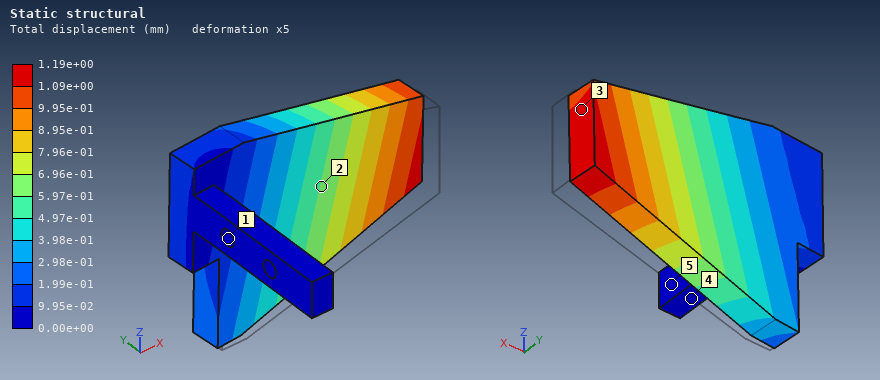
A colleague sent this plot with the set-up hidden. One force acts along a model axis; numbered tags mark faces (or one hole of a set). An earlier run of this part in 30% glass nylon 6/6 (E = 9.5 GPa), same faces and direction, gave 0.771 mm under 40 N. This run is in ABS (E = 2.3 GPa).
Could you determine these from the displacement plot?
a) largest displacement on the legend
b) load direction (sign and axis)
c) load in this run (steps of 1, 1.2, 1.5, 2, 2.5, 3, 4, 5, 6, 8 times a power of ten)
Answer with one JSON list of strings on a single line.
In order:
["1.19e+00 mm", "+Y", "15 N"]
